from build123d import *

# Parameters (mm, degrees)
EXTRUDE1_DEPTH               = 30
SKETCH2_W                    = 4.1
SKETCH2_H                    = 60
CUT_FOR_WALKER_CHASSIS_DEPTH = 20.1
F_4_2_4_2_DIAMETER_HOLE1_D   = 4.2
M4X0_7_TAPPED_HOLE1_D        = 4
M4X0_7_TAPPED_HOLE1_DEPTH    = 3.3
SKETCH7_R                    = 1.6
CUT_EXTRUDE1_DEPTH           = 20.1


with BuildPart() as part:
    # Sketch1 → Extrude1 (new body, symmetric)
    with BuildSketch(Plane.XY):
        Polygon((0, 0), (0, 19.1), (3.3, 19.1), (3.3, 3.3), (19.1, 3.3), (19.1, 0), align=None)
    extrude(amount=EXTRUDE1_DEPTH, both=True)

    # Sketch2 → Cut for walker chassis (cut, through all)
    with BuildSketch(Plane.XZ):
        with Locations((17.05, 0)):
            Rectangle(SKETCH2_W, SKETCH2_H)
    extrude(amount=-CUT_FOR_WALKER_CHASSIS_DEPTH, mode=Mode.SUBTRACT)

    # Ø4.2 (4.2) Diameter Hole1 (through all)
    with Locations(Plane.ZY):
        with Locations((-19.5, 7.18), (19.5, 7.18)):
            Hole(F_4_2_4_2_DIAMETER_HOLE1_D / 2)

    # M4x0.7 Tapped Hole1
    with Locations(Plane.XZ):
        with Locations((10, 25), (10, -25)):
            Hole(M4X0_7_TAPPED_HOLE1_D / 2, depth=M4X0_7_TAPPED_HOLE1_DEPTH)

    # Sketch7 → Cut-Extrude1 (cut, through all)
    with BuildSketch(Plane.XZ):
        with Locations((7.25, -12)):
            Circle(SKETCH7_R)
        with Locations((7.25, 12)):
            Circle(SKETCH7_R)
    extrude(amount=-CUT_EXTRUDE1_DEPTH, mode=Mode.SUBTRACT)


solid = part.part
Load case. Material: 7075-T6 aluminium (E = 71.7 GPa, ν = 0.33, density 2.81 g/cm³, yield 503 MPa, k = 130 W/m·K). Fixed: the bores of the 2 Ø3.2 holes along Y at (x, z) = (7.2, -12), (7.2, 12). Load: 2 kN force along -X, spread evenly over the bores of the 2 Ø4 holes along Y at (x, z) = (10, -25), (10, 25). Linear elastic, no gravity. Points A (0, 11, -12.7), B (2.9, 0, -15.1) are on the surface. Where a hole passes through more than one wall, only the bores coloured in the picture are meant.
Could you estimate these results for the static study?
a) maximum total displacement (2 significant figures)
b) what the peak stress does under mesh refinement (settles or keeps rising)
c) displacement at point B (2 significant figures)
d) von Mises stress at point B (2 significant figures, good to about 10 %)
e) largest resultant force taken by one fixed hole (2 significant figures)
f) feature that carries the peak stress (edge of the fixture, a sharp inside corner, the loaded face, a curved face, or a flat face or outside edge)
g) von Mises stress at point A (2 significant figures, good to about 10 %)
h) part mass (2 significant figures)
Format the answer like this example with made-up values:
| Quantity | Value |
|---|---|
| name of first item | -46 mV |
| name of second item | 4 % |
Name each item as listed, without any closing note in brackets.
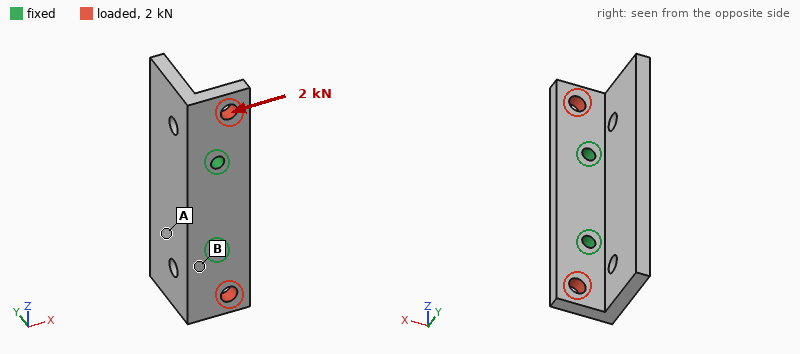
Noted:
| Quantity | Value |
|---|---|
| maximum total displacement | 53 µm |
| what the peak stress does under mesh refinement | keeps rising |
| displacement at point B | 9.4 µm |
| von Mises stress at point B | 50 MPa |
| largest resultant force taken by one fixed hole | 1.0 kN |
| feature that carries the peak stress | edge of the fixture |
| von Mises stress at point A | 20 MPa |
| part mass | 16 g |
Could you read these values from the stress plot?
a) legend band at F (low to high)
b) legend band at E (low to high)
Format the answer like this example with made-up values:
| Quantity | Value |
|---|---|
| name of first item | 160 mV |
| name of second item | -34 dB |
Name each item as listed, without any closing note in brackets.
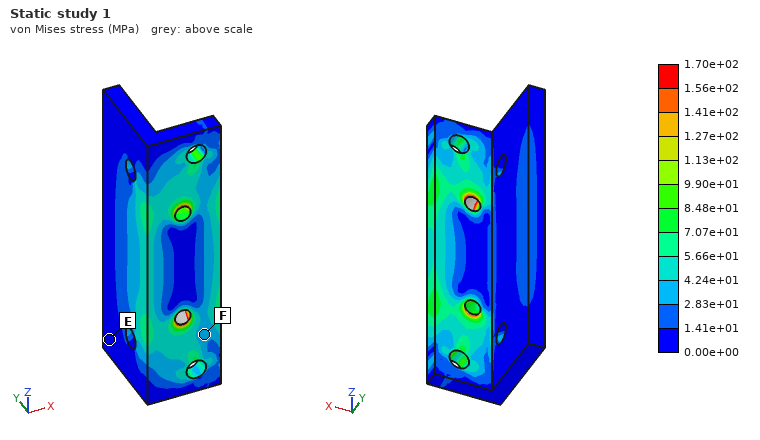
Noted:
| Quantity | Value |
|---|---|
| legend band at F | 2.83e+01 to 4.24e+01 MPa |
| legend band at E | 0.00e+00 to 1.41e+01 MPa |
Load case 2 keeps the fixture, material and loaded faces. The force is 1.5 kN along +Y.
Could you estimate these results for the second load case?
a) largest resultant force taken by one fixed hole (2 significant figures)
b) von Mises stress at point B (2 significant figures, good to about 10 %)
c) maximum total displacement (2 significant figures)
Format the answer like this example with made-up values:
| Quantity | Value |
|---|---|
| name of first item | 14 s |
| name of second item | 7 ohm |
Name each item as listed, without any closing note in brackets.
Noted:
| Quantity | Value |
|---|---|
| largest resultant force taken by one fixed hole | 810 N |
| von Mises stress at point B | 78 MPa |
| maximum total displacement | 0.15 mm |
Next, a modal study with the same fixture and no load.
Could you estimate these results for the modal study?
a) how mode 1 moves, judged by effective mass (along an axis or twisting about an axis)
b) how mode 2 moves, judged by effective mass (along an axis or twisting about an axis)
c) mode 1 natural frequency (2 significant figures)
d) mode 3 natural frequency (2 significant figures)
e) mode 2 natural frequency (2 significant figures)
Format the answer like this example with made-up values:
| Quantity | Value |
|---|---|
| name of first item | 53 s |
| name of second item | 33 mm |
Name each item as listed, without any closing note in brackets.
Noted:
| Quantity | Value |
|---|---|
| how mode 1 moves, judged by effective mass | along X |
| how mode 2 moves, judged by effective mass | twisting about Y |
| mode 1 natural frequency | 5200 Hz |
| mode 3 natural frequency | 11 kHz |
| mode 2 natural frequency | 6400 Hz |
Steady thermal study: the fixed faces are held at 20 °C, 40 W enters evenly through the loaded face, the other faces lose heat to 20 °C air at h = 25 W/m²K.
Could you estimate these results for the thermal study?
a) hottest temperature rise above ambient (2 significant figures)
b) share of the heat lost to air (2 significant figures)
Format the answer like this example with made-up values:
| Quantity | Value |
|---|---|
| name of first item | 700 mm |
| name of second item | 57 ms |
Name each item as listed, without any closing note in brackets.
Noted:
| Quantity | Value |
|---|---|
| hottest temperature rise above ambient | 48 K |
| share of the heat lost to air | 4.1 % |
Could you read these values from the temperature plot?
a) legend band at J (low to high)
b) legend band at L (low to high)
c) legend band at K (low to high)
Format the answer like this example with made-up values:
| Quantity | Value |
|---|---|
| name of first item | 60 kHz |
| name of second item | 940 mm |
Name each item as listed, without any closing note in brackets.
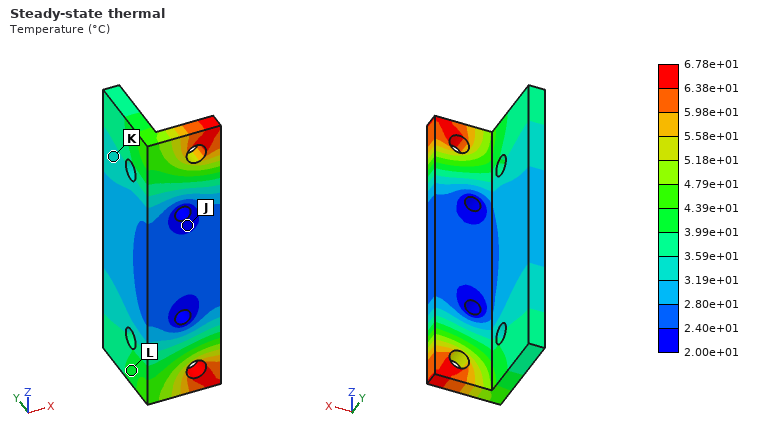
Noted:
| Quantity | Value |
|---|---|
| legend band at J | 2.00e+01 to 2.40e+01 °C |
| legend band at L | 3.99e+01 to 4.39e+01 °C |
| legend band at K | 3.19e+01 to 3.59e+01 °C |
